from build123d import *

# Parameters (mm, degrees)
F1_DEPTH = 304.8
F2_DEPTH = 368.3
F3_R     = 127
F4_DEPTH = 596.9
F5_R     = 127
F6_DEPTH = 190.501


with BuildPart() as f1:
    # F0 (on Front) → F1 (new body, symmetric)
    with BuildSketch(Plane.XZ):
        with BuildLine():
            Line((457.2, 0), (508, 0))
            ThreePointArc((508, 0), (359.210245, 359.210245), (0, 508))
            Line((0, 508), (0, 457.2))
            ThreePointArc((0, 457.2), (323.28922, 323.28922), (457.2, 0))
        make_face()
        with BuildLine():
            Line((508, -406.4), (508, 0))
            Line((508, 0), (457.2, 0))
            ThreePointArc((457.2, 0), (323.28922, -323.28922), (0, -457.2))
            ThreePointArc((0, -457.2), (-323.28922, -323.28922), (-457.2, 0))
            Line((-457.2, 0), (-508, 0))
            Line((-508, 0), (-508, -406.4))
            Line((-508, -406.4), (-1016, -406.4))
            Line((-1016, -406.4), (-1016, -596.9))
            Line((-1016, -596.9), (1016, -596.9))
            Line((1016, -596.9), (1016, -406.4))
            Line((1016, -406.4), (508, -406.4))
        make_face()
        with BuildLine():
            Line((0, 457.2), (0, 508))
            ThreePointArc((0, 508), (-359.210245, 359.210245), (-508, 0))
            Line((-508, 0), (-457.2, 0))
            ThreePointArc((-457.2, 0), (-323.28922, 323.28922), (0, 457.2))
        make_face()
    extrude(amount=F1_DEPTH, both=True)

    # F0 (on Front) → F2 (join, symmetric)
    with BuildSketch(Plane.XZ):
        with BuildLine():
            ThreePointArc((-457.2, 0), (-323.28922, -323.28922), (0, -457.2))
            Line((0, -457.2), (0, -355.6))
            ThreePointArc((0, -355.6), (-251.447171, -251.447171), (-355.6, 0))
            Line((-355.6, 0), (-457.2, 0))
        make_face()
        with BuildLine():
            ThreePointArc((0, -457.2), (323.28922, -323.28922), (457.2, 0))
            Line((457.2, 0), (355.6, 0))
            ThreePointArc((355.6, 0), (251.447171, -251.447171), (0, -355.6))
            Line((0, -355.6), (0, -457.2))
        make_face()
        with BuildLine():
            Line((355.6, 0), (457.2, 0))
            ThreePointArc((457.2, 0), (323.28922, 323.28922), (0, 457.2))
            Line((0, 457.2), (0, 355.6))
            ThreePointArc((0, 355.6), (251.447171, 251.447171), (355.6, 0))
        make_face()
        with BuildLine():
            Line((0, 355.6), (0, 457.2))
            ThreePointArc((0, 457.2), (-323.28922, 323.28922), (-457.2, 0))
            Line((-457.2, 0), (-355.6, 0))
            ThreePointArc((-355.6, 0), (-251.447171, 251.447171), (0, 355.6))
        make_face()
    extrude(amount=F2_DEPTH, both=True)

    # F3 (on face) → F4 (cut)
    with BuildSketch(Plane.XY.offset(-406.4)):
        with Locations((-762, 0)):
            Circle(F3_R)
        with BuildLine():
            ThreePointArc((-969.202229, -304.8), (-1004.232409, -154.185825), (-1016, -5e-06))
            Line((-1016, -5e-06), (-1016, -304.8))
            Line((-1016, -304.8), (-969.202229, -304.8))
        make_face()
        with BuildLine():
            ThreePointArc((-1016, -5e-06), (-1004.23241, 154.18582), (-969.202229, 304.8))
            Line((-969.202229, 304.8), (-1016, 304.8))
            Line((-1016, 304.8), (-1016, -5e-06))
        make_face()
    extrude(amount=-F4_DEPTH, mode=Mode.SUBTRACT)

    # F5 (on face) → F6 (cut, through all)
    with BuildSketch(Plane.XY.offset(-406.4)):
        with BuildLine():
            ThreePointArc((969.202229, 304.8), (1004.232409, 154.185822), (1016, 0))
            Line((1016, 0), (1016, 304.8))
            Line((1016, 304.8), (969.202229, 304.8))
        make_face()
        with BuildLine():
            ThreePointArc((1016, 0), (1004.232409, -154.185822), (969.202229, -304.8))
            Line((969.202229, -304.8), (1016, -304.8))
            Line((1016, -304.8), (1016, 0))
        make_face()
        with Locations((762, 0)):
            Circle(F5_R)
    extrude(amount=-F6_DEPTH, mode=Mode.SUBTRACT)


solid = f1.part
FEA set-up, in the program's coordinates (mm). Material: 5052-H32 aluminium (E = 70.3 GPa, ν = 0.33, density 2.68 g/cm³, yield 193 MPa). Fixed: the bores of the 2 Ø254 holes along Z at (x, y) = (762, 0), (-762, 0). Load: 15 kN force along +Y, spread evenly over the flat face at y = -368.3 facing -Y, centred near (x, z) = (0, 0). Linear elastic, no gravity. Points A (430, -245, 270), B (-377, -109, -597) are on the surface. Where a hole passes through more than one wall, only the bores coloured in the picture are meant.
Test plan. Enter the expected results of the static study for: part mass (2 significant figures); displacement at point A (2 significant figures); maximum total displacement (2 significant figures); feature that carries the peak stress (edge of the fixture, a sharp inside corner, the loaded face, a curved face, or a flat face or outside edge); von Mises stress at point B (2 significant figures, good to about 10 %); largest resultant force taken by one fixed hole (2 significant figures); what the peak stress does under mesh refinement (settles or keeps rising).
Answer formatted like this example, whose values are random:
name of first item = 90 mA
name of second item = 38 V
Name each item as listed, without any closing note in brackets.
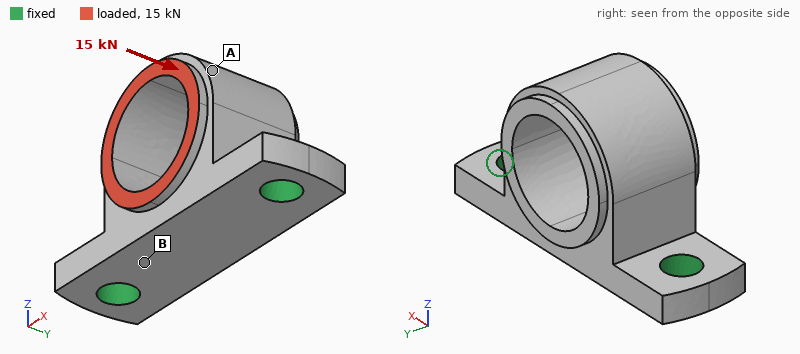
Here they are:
part mass = 1300 kg
displacement at point A = 20 µm
maximum total displacement = 26 µm
feature that carries the peak stress = edge of the fixture
von Mises stress at point B = 0.20 MPa
largest resultant force taken by one fixed hole = 7.5 kN
what the peak stress does under mesh refinement = keeps rising
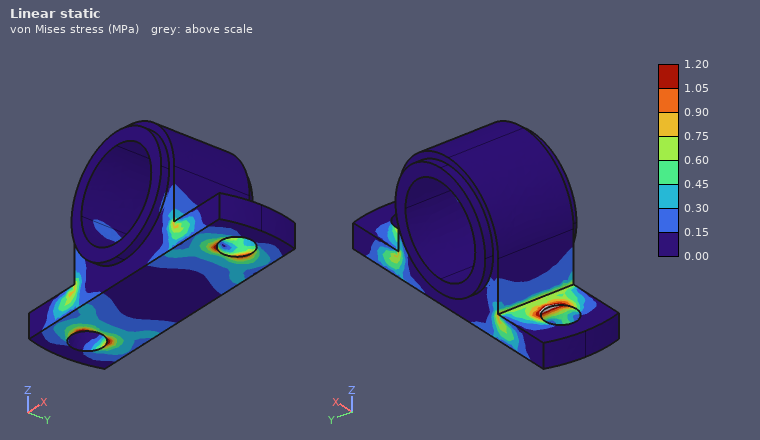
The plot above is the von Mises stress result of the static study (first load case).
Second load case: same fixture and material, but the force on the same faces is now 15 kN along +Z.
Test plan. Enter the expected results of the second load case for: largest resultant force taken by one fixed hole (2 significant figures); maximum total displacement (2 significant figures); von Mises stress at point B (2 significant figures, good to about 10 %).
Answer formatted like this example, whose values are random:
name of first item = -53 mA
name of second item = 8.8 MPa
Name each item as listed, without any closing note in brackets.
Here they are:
largest resultant force taken by one fixed hole = 8.0 kN
maximum total displacement = 20 µm
von Mises stress at point B = 0.23 MPa
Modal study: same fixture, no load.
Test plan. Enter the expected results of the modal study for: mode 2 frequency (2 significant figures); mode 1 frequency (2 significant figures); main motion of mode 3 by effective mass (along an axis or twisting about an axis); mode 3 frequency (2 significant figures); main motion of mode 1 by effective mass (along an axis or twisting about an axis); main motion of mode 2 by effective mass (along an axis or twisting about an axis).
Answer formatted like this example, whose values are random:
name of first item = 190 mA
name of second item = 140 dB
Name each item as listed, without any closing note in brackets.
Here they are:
mode 2 frequency = 290 Hz
mode 1 frequency = 160 Hz
main motion of mode 3 by effective mass = along Z
mode 3 frequency = 420 Hz
main motion of mode 1 by effective mass = along Y
main motion of mode 2 by effective mass = along X
